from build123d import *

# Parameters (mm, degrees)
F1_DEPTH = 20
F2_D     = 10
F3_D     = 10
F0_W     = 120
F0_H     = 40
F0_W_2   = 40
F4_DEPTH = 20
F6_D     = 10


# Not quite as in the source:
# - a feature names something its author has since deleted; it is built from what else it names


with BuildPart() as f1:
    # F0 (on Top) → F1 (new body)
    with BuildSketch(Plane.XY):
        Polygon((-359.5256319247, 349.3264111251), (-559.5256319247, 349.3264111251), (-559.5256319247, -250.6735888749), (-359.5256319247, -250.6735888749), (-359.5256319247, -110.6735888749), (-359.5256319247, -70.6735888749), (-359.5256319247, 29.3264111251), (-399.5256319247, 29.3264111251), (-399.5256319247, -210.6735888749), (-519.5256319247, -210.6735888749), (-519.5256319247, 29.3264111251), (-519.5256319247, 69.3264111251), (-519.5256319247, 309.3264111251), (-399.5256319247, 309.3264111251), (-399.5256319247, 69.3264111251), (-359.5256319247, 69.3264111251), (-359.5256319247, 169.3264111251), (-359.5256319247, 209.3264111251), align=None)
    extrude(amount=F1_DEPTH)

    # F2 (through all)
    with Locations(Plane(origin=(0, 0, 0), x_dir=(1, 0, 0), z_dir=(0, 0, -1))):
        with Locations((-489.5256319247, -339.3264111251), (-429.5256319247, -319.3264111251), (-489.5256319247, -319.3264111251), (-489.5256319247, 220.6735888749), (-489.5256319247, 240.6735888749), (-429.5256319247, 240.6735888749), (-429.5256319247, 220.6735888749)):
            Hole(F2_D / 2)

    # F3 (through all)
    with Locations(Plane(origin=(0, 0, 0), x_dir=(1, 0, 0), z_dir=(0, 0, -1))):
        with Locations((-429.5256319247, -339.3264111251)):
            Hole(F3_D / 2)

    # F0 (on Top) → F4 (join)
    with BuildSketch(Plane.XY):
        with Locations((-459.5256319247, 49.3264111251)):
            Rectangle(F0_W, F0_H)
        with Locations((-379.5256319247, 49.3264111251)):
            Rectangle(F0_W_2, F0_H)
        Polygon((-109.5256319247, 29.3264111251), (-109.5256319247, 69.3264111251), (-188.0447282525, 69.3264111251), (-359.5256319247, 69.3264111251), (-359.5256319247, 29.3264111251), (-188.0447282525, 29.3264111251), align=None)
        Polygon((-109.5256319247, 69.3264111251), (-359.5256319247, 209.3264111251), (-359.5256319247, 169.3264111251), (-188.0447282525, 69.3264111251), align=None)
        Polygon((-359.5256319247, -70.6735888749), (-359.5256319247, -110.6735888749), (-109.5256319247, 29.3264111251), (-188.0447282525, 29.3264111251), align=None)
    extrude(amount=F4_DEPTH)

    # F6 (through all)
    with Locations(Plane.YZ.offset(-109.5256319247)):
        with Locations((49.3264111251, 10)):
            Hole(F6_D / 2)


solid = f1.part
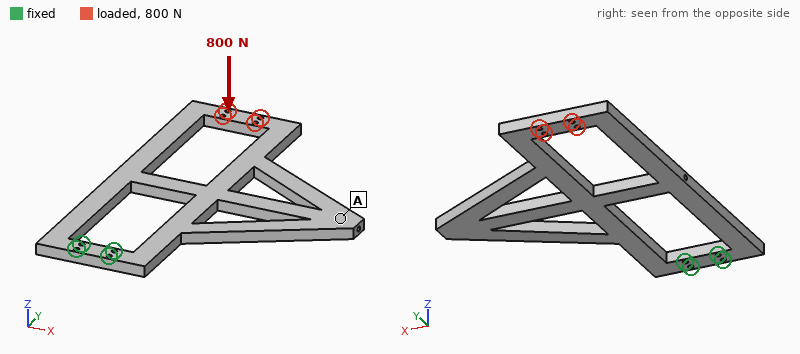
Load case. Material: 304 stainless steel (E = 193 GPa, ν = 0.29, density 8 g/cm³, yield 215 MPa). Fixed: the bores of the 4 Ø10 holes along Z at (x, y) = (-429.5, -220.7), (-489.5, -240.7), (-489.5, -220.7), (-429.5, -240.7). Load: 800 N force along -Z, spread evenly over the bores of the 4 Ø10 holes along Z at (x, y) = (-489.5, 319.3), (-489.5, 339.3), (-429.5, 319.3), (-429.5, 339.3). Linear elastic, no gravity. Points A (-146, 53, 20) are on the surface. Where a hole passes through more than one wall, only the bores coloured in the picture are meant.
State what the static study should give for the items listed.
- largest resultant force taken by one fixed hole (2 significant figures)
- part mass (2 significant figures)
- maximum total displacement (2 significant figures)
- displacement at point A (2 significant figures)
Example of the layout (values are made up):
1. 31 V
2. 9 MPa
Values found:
1. 6.2 kN
2. 14 kg
3. 5.0 mm
4. 1.7 mm
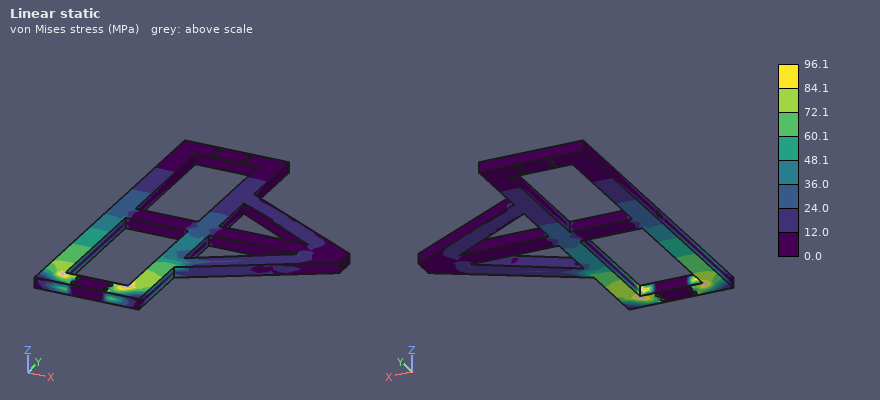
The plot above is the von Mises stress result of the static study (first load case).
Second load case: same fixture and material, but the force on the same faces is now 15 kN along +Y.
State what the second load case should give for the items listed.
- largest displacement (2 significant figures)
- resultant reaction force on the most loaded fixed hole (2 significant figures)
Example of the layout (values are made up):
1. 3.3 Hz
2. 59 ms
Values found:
1. 75 µm
2. 10 kN
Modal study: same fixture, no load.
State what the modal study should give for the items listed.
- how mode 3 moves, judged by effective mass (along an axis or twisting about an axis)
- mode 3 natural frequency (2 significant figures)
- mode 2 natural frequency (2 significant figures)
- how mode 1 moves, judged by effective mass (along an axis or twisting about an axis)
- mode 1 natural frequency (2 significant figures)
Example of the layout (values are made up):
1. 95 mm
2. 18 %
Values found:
1. along X
2. 130 Hz
3. 81 Hz
4. along Z
5. 34 Hz
